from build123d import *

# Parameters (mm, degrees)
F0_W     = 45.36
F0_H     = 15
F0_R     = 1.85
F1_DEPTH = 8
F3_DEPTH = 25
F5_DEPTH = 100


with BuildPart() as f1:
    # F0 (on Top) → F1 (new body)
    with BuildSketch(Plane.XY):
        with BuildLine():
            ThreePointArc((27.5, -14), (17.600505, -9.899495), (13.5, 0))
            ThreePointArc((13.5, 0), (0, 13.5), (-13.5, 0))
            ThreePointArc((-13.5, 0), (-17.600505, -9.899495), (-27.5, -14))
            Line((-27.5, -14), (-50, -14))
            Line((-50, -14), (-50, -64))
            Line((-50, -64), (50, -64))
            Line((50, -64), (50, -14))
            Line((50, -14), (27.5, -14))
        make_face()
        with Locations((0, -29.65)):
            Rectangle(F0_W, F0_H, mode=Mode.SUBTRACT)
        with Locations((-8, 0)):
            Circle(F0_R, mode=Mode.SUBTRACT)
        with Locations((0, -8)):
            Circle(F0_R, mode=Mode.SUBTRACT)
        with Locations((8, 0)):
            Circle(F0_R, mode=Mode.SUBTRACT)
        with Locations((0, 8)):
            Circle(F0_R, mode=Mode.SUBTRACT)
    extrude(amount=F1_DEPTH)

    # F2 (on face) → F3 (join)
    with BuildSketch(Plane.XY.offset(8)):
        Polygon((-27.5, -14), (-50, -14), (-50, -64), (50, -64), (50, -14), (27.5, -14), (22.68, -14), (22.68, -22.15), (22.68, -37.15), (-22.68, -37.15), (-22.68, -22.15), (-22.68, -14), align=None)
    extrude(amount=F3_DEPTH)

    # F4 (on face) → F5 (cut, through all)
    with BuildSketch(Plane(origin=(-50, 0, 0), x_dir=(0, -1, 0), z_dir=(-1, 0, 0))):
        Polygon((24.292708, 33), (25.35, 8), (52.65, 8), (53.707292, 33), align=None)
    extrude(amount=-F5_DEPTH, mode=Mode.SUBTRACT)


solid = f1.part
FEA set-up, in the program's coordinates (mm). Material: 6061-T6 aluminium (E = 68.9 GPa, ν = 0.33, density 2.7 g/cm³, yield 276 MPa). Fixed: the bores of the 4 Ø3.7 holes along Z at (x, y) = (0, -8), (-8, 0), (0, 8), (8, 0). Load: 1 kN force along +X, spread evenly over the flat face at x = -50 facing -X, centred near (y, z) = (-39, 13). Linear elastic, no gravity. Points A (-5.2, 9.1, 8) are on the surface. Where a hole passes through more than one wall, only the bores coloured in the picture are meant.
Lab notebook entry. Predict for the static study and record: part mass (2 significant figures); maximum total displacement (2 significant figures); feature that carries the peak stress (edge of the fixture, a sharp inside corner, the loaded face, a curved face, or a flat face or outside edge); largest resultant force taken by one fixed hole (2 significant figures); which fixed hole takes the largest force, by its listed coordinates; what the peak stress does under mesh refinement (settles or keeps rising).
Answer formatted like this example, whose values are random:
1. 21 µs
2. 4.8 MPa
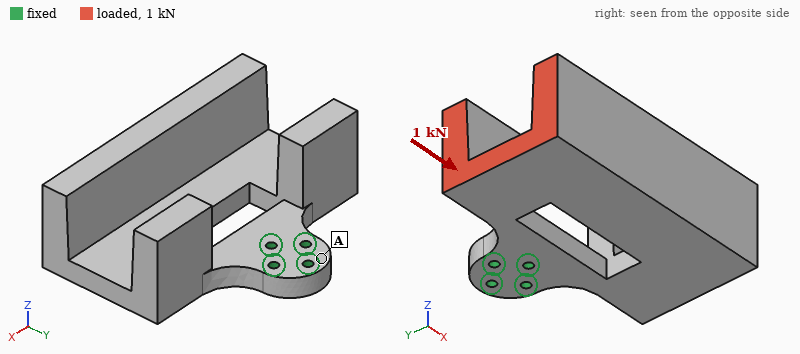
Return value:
1. 220 g
2. 0.16 mm
3. edge of the fixture
4. 1.8 kN
5. (0, -8)
6. keeps rising
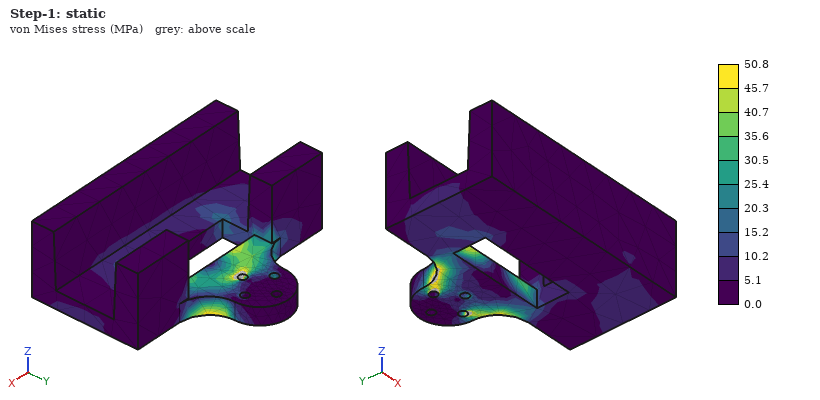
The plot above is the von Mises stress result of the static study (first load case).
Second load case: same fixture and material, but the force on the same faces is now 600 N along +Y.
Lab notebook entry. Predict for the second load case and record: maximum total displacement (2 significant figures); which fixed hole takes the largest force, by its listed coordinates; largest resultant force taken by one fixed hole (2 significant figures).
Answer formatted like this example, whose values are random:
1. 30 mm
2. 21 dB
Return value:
1. 0.19 mm
2. (-8, 0)
3. 1.5 kN
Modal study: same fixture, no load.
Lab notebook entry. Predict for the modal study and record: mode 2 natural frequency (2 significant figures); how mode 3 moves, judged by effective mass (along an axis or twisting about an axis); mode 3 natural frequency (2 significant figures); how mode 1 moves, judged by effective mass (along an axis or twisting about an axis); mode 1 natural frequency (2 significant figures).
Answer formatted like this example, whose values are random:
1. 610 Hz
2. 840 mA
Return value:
1. 760 Hz
2. along X
3. 1300 Hz
4. along Z
5. 490 Hz
